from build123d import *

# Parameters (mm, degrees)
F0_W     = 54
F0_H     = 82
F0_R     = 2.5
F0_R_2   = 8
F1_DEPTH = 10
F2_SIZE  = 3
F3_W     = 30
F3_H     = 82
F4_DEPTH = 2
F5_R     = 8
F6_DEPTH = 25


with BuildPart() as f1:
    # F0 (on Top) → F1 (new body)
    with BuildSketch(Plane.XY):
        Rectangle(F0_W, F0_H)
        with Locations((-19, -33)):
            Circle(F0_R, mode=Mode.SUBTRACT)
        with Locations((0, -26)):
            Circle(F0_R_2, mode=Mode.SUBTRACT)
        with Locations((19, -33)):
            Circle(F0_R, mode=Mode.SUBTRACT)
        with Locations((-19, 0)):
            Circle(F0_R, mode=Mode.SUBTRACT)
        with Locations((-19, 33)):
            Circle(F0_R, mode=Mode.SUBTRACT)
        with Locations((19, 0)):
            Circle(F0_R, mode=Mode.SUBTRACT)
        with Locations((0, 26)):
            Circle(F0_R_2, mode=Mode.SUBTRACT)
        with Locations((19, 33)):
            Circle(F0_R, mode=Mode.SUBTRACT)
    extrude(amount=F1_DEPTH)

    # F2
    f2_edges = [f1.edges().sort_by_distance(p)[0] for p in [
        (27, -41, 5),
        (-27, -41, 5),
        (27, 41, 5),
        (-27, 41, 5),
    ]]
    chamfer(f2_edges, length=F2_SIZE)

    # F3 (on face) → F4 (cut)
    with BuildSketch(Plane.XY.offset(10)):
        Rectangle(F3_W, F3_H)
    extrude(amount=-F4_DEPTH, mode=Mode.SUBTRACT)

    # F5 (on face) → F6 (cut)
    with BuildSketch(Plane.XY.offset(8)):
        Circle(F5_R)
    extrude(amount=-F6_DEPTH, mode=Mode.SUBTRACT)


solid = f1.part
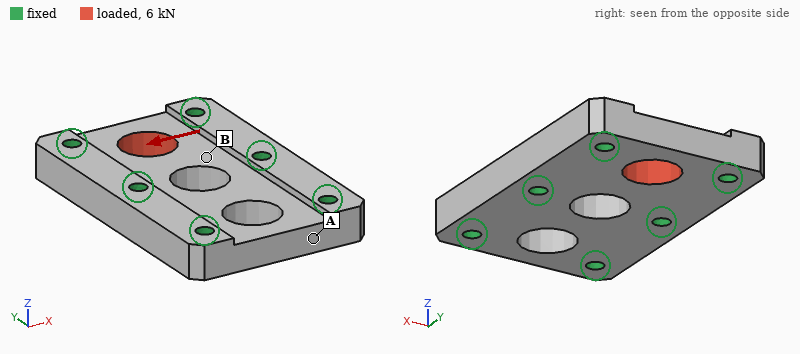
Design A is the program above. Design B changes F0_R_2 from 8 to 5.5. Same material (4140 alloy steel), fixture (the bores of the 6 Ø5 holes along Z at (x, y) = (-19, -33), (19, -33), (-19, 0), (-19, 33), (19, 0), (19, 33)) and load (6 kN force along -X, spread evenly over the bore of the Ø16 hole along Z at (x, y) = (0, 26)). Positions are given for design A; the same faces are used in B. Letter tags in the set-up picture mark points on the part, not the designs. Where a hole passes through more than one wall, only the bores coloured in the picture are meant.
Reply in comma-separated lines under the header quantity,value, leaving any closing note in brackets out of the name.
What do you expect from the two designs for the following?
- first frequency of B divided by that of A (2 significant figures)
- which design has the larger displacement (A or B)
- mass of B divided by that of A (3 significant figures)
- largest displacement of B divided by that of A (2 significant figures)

quantity,value
first frequency of B divided by that of A,0.97
which design has the larger displacement,B
mass of B divided by that of A,1.05
largest displacement of B divided by that of A,1.2
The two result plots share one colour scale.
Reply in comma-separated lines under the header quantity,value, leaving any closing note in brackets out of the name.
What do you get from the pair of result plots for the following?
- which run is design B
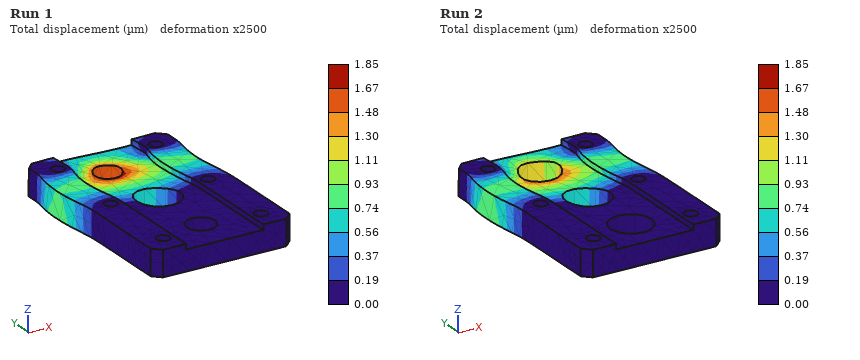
quantity,value
which run is design B,Run 1
